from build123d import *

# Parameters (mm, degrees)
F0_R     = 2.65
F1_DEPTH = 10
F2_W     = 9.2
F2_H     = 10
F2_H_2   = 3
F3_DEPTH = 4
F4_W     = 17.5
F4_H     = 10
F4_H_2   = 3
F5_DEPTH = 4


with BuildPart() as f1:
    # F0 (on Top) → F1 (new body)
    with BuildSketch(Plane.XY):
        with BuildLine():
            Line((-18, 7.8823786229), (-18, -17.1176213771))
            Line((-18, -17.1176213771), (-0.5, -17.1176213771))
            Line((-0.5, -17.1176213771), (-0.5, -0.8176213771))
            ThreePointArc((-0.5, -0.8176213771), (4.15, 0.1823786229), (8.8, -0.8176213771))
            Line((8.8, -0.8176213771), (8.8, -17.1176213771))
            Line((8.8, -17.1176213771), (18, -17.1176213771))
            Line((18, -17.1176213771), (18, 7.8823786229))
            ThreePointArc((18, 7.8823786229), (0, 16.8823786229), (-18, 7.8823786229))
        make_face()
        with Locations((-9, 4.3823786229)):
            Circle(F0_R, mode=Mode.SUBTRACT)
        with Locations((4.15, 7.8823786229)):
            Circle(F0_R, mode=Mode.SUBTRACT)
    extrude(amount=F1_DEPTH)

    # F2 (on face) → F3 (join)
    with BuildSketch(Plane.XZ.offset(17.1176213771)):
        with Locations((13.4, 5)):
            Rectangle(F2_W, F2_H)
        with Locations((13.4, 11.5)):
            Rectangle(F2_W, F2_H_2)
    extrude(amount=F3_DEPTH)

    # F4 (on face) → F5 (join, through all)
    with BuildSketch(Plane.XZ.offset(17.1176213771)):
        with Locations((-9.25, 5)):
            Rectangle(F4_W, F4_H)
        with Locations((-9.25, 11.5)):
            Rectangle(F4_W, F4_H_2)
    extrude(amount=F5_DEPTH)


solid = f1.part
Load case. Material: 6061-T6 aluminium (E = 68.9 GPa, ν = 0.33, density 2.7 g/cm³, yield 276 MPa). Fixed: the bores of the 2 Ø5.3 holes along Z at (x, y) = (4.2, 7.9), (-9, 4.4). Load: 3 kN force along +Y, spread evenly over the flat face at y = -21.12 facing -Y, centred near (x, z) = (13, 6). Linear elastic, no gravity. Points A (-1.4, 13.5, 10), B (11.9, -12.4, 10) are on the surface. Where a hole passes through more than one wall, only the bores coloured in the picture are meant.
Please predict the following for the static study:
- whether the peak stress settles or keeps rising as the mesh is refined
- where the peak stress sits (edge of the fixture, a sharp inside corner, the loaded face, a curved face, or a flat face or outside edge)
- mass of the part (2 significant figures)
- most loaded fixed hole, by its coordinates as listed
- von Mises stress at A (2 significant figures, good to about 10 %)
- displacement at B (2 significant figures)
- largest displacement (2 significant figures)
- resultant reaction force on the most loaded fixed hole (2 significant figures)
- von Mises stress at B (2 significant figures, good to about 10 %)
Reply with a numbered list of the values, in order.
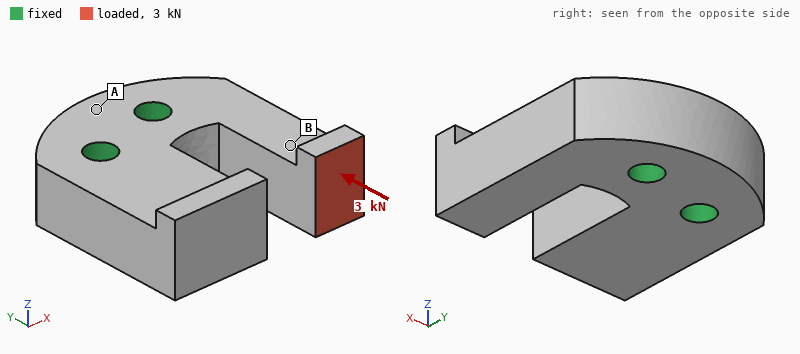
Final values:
1. keeps rising
2. edge of the fixture
3. 29 g
4. (4.2, 7.9)
5. 13 MPa
6. 45 µm
7. 83 µm
8. 3.8 kN
9. 63 MPa
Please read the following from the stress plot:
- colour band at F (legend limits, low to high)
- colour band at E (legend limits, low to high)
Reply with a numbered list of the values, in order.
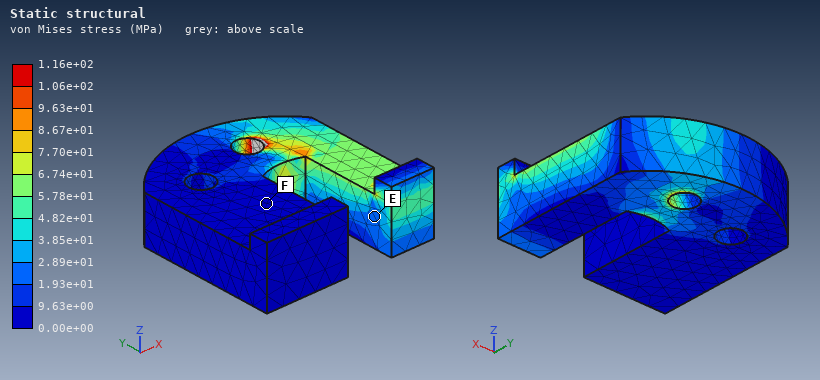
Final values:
1. 0.00e+00 to 9.63e+00 MPa
2. 1.93e+01 to 2.89e+01 MPa
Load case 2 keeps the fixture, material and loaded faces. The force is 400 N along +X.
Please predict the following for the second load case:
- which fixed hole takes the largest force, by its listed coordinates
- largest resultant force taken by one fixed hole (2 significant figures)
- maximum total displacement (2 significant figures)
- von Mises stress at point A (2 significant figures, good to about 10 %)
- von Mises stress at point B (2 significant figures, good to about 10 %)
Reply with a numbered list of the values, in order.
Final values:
1. (-9, 4.4)
2. 420 N
3. 72 µm
4. 5.6 MPa
5. 19 MPa
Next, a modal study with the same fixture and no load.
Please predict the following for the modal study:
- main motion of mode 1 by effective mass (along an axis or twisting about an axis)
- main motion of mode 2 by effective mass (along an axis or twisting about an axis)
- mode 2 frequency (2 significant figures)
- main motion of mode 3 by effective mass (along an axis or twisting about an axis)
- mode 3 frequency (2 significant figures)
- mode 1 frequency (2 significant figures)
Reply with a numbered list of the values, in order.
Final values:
1. along Z
2. along X
3. 8600 Hz
4. along Z
5. 11 kHz
6. 7900 Hz
